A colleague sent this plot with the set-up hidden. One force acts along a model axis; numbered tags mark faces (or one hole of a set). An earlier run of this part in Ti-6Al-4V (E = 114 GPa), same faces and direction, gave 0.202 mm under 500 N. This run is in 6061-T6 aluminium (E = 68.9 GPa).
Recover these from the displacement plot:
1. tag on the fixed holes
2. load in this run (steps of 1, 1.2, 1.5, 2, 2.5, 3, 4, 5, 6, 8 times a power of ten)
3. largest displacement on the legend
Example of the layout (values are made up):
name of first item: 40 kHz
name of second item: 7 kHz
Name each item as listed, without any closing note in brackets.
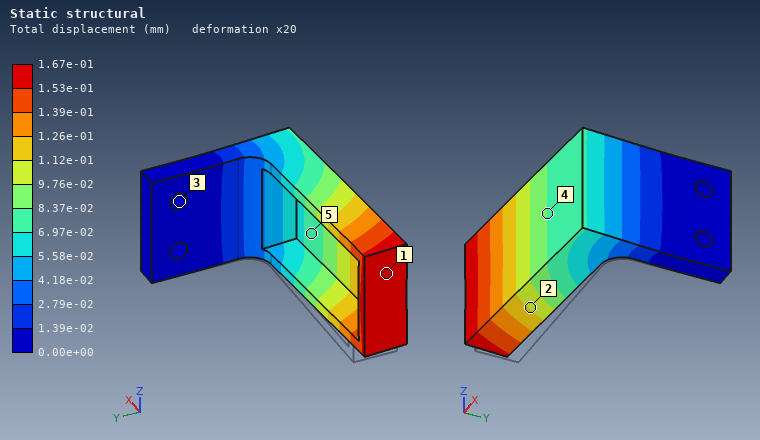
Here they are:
tag on the fixed holes: 3
load in this run: 250 N
largest displacement on the legend: 1.67e-01 mm
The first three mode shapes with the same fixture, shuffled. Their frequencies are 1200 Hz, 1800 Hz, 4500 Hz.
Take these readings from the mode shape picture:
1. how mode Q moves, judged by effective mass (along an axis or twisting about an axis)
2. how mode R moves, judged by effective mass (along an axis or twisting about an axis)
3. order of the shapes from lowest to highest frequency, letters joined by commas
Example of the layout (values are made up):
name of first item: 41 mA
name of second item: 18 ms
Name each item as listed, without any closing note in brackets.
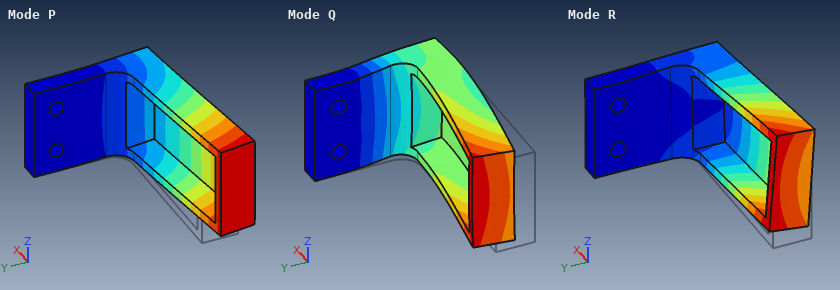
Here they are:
how mode Q moves, judged by effective mass: along X
how mode R moves, judged by effective mass: along Z
order of the shapes from lowest to highest frequency, letters joined by commas: P, R, Q
